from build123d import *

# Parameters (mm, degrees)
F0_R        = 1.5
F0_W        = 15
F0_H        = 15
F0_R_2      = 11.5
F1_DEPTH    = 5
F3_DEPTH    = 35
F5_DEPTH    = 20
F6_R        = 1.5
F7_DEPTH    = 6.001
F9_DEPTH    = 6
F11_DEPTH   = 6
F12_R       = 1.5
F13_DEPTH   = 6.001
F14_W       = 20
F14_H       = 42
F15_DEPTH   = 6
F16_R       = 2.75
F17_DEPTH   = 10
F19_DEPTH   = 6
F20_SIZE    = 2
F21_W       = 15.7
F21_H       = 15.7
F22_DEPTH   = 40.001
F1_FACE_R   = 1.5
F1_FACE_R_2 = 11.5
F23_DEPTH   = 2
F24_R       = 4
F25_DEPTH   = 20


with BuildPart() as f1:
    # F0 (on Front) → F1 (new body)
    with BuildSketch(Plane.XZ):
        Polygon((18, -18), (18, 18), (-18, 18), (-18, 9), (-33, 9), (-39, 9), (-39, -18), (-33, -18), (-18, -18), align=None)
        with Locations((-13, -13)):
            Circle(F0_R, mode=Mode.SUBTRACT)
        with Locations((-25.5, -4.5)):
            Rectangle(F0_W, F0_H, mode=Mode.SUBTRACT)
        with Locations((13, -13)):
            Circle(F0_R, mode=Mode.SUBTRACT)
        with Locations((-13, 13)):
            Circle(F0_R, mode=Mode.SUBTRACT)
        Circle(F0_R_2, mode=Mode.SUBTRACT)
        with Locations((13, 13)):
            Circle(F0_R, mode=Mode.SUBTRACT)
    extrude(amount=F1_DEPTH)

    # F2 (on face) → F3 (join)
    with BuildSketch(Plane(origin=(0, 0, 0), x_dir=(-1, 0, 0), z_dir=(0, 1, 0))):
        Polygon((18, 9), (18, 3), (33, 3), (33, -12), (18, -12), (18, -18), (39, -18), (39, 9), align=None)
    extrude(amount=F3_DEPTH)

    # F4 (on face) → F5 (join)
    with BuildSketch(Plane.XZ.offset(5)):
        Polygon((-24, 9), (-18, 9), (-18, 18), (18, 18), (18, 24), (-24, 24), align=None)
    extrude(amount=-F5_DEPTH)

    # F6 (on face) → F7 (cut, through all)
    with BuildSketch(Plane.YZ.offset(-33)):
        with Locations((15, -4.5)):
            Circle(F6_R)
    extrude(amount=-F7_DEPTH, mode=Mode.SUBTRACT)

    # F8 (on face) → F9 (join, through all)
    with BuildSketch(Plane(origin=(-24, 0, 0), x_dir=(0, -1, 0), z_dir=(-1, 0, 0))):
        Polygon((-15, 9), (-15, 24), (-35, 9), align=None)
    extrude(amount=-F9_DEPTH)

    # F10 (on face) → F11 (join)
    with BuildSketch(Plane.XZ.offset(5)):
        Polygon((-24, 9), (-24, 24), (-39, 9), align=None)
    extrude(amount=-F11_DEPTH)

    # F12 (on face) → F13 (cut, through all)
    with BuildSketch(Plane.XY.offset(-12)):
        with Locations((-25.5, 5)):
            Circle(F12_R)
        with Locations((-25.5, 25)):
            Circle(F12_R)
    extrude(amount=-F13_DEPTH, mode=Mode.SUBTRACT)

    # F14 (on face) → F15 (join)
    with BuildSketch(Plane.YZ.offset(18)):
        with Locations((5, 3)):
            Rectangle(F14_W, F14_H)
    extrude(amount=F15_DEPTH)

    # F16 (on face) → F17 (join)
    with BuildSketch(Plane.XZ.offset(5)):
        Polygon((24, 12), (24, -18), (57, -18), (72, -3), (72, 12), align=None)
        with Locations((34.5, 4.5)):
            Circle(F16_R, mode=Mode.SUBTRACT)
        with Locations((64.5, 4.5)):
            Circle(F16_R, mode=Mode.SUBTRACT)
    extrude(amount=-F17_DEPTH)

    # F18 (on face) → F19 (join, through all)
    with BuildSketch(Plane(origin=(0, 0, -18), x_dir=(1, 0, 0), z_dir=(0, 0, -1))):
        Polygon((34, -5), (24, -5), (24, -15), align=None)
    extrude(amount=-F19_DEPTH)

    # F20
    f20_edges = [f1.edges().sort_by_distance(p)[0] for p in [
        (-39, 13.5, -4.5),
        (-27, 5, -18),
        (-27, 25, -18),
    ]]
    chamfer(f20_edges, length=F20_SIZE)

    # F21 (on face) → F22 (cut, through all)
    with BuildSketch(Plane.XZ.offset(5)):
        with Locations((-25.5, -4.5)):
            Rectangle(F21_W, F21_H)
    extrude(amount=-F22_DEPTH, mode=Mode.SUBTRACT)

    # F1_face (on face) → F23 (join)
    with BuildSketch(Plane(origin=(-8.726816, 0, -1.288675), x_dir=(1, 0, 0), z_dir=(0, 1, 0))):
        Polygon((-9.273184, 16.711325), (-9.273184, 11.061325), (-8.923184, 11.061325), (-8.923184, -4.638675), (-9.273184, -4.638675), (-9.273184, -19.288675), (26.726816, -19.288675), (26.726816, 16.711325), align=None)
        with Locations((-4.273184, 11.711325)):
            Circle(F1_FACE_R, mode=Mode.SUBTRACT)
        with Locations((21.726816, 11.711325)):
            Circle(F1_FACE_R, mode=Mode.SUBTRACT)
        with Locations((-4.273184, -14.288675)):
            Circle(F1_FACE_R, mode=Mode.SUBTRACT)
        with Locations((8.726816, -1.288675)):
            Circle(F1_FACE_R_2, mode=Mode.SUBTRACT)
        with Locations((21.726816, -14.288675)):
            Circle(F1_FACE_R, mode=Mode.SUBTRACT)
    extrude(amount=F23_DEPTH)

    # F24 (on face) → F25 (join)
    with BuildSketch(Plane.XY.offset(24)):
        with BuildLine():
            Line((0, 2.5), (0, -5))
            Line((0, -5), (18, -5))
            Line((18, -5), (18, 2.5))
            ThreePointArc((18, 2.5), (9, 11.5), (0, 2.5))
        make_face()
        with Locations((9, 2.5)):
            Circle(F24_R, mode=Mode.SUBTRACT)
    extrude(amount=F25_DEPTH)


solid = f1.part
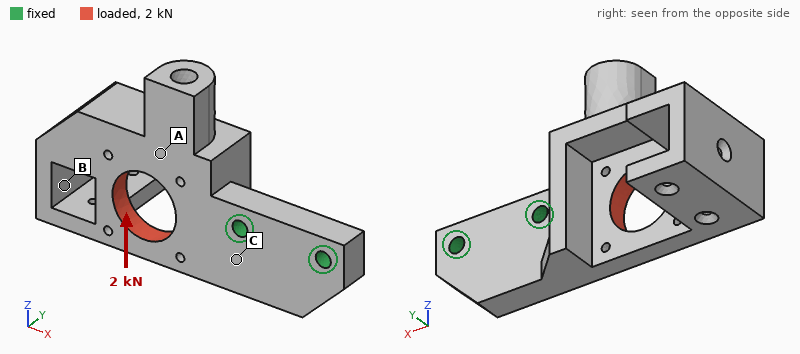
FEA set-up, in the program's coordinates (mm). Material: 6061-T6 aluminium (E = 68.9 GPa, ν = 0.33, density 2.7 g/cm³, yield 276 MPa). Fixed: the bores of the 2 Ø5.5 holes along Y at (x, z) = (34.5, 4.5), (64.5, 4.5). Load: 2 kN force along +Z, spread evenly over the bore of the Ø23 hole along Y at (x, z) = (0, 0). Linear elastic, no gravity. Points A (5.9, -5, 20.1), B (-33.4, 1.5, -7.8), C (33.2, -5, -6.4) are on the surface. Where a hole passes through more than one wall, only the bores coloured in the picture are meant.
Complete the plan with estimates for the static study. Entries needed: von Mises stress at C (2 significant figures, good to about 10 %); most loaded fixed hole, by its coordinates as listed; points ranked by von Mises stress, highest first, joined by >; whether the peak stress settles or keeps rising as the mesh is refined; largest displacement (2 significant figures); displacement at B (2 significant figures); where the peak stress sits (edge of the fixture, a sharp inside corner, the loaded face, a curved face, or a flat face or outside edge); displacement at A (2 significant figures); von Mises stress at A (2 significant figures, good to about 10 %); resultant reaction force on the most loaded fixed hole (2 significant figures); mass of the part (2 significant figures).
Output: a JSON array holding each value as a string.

["20 MPa", "(34.5, 4.5)", "C > A > B", "keeps rising", "0.15 mm", "0.13 mm", "edge of the fixture", "0.063 mm", "13 MPa", "4.0 kN", "130 g"]
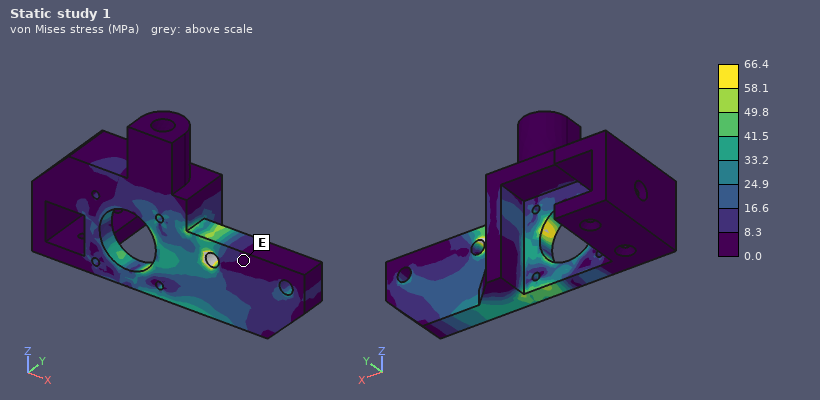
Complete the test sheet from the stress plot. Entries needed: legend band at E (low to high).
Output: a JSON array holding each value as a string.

["0.0 to 8.3 MPa"]
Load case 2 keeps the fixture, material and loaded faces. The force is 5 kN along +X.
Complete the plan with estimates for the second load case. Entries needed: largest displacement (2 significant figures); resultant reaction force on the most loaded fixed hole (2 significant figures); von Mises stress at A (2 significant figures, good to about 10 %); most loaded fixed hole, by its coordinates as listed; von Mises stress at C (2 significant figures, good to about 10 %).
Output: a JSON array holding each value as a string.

["67 µm", "4.2 kN", "9.4 MPa", "(34.5, 4.5)", "19 MPa"]
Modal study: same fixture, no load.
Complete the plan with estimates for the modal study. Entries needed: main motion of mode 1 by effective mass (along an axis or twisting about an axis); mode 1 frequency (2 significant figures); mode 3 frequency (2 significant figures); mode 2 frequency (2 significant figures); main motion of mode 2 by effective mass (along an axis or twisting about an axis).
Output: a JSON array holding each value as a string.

["along Y", "830 Hz", "2500 Hz", "1400 Hz", "along Z"]
